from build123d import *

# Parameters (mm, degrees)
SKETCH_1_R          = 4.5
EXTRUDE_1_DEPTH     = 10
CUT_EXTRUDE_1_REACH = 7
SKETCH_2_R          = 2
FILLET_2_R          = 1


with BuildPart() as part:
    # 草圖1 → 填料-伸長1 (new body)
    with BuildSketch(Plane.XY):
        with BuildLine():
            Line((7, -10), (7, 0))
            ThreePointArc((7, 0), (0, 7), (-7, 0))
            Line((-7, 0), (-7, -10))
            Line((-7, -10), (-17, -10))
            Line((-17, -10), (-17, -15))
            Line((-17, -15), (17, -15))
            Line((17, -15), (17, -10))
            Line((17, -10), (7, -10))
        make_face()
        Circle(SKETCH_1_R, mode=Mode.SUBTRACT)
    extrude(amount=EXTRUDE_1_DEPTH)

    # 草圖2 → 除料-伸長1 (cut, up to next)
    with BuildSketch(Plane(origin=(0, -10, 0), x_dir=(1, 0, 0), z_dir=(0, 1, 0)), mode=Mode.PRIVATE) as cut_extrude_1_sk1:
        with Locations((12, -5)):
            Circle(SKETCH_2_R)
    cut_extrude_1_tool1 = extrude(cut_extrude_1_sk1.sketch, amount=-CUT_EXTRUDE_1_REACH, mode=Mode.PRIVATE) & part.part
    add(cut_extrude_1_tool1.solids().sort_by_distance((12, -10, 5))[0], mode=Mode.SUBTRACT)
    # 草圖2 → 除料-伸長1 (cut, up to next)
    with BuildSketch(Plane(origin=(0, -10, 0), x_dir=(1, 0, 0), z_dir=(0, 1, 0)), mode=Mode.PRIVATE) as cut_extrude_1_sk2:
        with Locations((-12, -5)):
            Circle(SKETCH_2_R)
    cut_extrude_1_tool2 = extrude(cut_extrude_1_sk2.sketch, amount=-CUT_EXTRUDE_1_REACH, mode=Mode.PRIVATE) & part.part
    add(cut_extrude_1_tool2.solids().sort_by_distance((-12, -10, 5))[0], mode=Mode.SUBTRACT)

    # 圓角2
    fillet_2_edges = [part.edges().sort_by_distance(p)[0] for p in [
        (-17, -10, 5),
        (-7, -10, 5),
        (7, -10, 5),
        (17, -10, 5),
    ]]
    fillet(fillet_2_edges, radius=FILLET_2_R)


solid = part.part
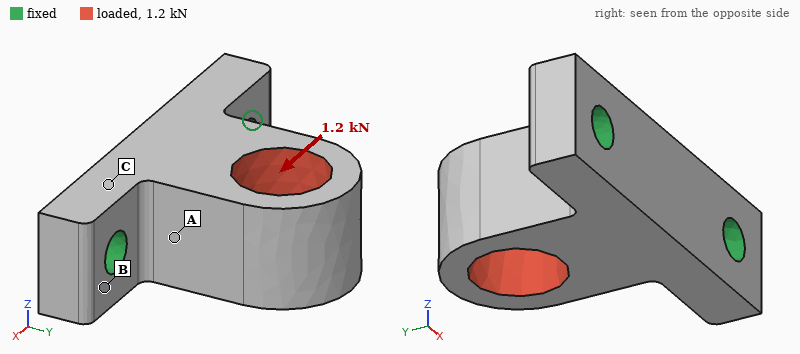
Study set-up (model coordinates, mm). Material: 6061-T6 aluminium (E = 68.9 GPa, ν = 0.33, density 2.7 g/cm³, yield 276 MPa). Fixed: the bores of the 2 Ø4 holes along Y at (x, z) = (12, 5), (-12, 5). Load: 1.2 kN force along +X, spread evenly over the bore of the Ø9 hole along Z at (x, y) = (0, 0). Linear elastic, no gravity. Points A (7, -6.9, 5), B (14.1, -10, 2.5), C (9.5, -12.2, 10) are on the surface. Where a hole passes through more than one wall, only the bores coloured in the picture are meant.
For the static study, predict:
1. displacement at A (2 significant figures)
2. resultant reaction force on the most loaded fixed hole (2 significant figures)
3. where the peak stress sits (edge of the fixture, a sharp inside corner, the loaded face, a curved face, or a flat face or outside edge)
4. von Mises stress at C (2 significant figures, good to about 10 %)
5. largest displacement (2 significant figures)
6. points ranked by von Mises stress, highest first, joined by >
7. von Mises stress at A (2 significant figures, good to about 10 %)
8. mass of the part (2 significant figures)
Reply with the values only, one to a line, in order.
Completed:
8.3 µm
1.0 kN
a curved face
30 MPa
38 µm
A > C > B
48 MPa
8.4 g
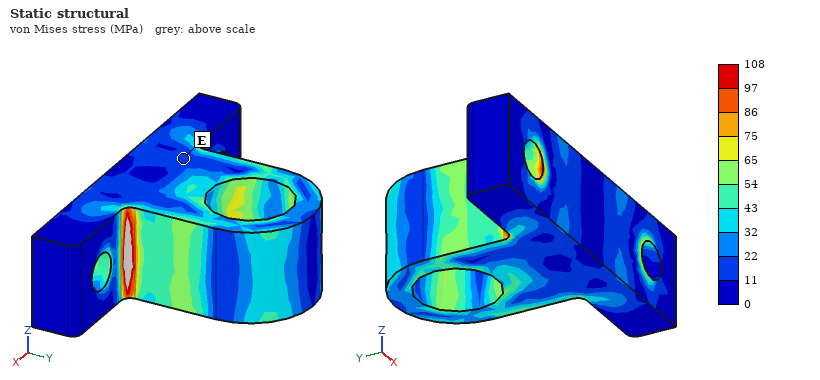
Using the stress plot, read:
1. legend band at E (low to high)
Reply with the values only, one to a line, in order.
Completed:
11 to 22 MPa
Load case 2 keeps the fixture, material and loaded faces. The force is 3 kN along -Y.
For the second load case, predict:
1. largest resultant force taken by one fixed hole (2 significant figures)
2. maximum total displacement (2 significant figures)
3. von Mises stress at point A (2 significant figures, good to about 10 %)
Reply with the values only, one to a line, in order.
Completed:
1.6 kN
24 µm
56 MPa
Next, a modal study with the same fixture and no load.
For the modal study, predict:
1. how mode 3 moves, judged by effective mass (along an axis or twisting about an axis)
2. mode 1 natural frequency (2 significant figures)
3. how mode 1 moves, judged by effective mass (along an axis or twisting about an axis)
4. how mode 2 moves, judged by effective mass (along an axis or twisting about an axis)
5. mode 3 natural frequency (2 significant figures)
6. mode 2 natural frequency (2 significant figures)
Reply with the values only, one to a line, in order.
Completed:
along Y
11 kHz
along Z
along X
31 kHz
20 kHz
